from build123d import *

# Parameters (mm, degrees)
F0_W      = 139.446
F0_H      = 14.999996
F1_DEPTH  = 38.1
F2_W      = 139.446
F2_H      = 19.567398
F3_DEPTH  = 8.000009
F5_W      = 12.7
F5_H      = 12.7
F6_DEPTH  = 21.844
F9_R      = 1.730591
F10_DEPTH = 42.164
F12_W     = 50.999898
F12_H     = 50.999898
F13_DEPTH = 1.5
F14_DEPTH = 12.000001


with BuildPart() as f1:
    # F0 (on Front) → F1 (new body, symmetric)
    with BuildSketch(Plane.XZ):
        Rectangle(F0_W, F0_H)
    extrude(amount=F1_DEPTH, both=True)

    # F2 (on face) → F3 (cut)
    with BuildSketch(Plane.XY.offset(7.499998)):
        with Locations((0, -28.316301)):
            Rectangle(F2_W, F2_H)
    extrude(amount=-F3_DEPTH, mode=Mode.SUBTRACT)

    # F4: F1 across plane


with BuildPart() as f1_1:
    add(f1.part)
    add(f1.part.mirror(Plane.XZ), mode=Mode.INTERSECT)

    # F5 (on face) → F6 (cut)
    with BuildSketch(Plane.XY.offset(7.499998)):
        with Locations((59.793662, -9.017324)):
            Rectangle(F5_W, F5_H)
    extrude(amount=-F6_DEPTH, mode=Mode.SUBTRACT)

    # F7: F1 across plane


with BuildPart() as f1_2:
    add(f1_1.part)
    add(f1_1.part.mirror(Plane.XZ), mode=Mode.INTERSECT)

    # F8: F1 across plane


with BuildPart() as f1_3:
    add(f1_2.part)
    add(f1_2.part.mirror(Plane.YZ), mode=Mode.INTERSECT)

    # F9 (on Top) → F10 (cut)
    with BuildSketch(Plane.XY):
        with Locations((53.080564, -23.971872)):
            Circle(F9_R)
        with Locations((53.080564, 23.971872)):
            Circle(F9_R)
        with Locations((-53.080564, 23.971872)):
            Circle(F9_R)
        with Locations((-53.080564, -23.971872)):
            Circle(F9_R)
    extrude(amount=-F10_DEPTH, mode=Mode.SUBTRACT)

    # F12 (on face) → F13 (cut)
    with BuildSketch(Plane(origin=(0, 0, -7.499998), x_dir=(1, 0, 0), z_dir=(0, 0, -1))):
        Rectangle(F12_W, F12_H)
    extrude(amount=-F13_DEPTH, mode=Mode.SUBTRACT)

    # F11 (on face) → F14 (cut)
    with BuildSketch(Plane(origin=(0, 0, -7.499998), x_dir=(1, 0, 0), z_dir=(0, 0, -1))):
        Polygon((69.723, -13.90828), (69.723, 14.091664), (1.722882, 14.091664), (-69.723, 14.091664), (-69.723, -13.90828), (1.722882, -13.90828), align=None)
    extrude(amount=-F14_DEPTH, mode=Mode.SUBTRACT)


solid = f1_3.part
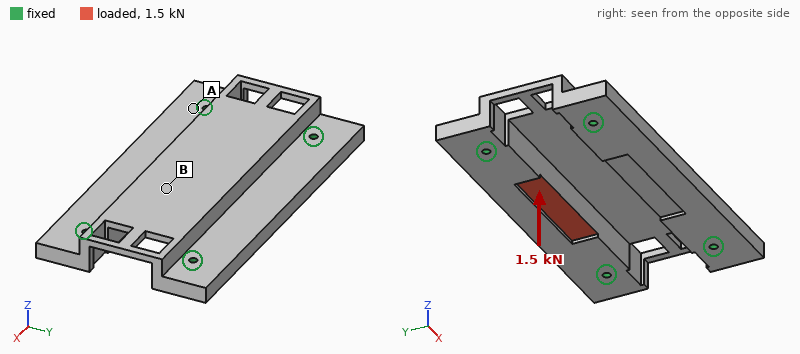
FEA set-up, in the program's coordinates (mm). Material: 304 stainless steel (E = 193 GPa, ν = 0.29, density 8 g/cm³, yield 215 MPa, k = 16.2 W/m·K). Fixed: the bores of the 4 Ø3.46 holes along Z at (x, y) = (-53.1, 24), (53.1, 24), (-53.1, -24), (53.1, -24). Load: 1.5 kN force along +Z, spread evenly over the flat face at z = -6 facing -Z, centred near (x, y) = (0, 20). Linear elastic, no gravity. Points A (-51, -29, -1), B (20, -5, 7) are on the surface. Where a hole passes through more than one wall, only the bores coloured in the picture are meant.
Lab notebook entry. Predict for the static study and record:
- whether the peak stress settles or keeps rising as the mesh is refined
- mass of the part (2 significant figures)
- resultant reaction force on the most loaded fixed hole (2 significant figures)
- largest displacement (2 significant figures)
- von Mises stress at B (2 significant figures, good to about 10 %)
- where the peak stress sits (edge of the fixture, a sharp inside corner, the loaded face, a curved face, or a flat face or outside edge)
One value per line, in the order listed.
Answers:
keeps rising
510 g
1.1 kN
30 µm
12 MPa
edge of the fixture
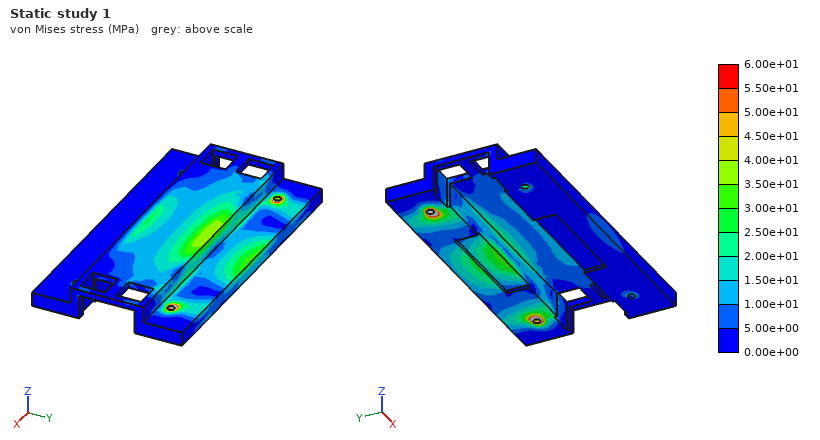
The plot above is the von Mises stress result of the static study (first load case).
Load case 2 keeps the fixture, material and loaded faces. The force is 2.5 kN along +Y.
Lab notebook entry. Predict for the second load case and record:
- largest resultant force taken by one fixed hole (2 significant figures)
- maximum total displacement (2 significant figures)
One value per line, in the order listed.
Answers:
1.1 kN
33 µm
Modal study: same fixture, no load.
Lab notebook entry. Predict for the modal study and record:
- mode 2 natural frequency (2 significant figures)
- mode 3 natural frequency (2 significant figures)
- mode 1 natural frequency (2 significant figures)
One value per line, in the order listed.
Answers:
3600 Hz
6300 Hz
3600 Hz
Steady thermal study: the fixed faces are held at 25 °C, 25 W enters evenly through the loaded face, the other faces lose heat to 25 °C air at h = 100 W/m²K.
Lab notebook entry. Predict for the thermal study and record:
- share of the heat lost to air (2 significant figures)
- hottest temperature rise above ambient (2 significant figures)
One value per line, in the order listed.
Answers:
87 %
57 K
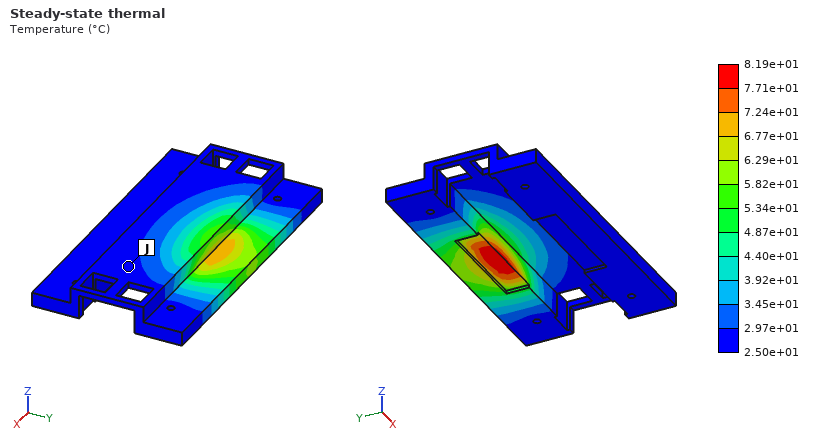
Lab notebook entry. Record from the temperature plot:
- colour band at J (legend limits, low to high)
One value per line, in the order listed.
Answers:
2.50e+01 to 2.97e+01 °C
